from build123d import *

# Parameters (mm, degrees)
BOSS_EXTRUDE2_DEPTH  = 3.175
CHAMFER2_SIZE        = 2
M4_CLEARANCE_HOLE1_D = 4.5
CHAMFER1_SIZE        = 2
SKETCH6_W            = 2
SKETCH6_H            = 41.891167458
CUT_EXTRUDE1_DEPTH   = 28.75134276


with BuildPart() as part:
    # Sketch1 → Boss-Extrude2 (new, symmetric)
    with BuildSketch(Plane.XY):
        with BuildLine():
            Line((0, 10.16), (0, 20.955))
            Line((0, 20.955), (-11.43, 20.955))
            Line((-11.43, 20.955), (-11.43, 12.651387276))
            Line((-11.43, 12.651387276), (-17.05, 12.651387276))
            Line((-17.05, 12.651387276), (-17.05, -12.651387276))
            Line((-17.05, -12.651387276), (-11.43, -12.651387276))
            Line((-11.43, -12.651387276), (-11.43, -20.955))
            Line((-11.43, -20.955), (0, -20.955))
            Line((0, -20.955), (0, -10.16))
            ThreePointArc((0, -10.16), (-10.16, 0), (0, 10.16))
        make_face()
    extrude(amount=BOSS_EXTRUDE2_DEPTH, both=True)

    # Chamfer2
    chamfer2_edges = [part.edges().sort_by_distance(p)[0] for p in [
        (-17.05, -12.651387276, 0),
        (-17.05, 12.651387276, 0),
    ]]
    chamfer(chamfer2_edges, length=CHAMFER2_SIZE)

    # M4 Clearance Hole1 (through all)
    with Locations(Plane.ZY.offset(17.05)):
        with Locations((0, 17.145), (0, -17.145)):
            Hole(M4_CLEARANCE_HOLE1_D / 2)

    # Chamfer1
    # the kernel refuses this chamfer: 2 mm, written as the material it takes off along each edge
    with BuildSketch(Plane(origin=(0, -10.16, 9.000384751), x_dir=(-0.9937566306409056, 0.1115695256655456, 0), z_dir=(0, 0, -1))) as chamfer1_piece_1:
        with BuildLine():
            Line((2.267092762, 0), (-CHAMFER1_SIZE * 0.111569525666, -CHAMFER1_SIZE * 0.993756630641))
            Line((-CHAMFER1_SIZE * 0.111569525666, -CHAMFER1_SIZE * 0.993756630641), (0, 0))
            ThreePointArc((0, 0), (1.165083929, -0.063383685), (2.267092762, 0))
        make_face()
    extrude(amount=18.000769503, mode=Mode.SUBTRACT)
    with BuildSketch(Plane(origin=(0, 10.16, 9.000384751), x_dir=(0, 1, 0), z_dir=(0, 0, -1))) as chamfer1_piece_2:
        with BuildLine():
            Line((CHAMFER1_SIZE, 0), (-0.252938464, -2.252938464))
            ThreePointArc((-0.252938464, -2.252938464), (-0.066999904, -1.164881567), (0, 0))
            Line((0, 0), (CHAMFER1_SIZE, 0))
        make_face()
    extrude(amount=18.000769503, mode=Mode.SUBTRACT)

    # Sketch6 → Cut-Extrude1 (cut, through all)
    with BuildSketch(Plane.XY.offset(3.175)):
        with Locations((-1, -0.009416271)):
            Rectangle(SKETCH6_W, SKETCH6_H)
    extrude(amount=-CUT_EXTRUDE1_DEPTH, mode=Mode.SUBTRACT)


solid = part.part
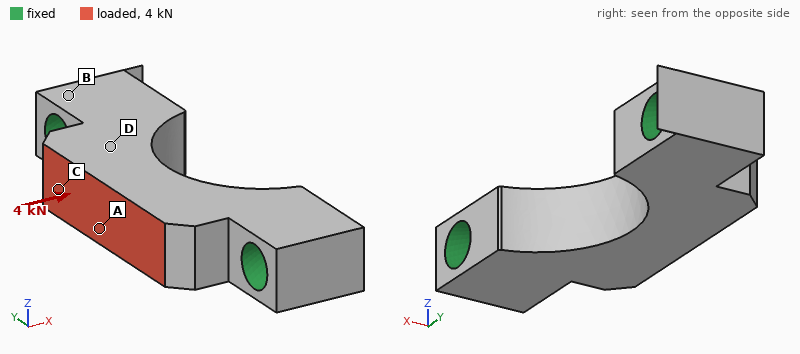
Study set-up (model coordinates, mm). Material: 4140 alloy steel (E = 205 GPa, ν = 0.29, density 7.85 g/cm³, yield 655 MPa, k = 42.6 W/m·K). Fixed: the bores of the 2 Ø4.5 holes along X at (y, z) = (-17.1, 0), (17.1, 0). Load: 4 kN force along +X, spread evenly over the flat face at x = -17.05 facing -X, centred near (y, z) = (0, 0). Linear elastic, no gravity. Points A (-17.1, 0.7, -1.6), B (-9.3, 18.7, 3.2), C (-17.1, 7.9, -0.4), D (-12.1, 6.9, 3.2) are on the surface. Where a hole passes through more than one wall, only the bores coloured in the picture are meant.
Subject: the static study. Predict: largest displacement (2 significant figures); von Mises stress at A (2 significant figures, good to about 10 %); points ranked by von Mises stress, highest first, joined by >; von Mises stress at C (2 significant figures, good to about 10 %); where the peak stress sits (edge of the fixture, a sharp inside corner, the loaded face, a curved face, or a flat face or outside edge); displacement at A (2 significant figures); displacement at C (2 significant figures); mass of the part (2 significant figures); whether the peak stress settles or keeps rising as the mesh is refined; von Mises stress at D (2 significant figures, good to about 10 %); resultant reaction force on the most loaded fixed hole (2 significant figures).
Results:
8.0 µm
80 MPa
A > D > C > B
31 MPa
edge of the fixture
7.9 µm
5.7 µm
18 g
keeps rising
54 MPa
2.5 kN
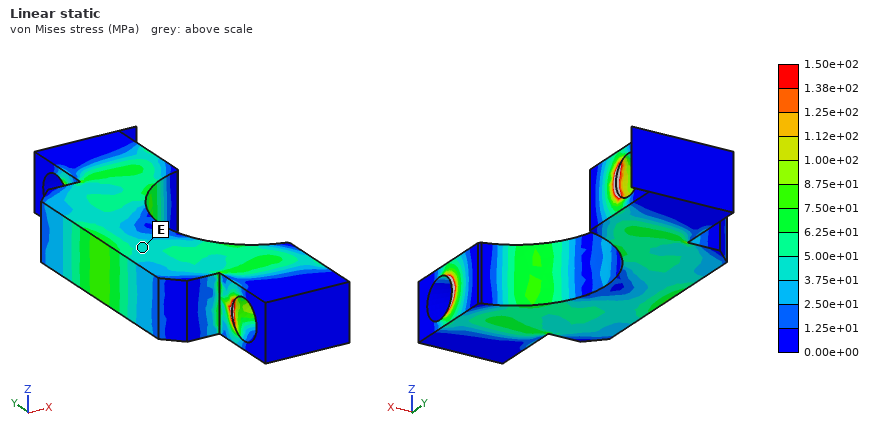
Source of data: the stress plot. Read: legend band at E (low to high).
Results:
3.75e+01 to 5.00e+01 MPa
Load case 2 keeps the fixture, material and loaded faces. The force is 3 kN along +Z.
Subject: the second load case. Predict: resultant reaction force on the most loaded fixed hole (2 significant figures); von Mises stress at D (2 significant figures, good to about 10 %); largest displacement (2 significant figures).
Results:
1.5 kN
140 MPa
49 µm
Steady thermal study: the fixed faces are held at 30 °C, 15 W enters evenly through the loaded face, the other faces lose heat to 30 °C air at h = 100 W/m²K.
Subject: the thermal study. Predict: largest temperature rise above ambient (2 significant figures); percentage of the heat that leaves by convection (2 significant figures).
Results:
44 K
13 %
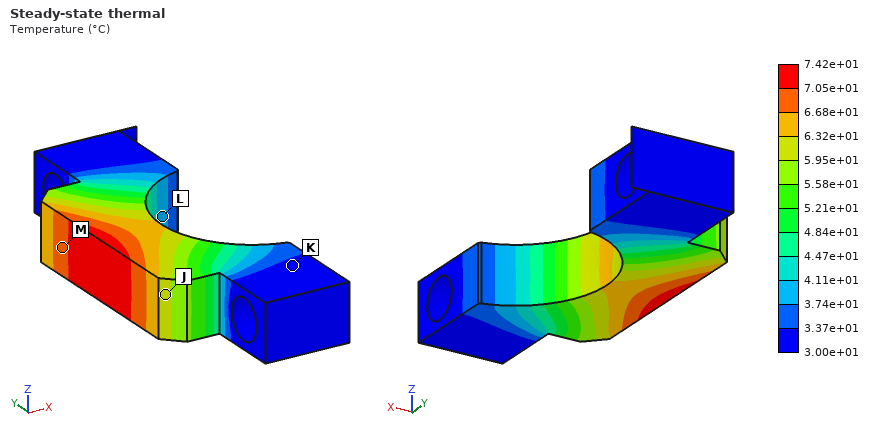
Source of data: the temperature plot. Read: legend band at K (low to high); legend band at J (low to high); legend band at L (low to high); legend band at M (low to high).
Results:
3.00e+01 to 3.37e+01 °C
5.95e+01 to 6.32e+01 °C
3.74e+01 to 4.11e+01 °C
6.68e+01 to 7.05e+01 °C
